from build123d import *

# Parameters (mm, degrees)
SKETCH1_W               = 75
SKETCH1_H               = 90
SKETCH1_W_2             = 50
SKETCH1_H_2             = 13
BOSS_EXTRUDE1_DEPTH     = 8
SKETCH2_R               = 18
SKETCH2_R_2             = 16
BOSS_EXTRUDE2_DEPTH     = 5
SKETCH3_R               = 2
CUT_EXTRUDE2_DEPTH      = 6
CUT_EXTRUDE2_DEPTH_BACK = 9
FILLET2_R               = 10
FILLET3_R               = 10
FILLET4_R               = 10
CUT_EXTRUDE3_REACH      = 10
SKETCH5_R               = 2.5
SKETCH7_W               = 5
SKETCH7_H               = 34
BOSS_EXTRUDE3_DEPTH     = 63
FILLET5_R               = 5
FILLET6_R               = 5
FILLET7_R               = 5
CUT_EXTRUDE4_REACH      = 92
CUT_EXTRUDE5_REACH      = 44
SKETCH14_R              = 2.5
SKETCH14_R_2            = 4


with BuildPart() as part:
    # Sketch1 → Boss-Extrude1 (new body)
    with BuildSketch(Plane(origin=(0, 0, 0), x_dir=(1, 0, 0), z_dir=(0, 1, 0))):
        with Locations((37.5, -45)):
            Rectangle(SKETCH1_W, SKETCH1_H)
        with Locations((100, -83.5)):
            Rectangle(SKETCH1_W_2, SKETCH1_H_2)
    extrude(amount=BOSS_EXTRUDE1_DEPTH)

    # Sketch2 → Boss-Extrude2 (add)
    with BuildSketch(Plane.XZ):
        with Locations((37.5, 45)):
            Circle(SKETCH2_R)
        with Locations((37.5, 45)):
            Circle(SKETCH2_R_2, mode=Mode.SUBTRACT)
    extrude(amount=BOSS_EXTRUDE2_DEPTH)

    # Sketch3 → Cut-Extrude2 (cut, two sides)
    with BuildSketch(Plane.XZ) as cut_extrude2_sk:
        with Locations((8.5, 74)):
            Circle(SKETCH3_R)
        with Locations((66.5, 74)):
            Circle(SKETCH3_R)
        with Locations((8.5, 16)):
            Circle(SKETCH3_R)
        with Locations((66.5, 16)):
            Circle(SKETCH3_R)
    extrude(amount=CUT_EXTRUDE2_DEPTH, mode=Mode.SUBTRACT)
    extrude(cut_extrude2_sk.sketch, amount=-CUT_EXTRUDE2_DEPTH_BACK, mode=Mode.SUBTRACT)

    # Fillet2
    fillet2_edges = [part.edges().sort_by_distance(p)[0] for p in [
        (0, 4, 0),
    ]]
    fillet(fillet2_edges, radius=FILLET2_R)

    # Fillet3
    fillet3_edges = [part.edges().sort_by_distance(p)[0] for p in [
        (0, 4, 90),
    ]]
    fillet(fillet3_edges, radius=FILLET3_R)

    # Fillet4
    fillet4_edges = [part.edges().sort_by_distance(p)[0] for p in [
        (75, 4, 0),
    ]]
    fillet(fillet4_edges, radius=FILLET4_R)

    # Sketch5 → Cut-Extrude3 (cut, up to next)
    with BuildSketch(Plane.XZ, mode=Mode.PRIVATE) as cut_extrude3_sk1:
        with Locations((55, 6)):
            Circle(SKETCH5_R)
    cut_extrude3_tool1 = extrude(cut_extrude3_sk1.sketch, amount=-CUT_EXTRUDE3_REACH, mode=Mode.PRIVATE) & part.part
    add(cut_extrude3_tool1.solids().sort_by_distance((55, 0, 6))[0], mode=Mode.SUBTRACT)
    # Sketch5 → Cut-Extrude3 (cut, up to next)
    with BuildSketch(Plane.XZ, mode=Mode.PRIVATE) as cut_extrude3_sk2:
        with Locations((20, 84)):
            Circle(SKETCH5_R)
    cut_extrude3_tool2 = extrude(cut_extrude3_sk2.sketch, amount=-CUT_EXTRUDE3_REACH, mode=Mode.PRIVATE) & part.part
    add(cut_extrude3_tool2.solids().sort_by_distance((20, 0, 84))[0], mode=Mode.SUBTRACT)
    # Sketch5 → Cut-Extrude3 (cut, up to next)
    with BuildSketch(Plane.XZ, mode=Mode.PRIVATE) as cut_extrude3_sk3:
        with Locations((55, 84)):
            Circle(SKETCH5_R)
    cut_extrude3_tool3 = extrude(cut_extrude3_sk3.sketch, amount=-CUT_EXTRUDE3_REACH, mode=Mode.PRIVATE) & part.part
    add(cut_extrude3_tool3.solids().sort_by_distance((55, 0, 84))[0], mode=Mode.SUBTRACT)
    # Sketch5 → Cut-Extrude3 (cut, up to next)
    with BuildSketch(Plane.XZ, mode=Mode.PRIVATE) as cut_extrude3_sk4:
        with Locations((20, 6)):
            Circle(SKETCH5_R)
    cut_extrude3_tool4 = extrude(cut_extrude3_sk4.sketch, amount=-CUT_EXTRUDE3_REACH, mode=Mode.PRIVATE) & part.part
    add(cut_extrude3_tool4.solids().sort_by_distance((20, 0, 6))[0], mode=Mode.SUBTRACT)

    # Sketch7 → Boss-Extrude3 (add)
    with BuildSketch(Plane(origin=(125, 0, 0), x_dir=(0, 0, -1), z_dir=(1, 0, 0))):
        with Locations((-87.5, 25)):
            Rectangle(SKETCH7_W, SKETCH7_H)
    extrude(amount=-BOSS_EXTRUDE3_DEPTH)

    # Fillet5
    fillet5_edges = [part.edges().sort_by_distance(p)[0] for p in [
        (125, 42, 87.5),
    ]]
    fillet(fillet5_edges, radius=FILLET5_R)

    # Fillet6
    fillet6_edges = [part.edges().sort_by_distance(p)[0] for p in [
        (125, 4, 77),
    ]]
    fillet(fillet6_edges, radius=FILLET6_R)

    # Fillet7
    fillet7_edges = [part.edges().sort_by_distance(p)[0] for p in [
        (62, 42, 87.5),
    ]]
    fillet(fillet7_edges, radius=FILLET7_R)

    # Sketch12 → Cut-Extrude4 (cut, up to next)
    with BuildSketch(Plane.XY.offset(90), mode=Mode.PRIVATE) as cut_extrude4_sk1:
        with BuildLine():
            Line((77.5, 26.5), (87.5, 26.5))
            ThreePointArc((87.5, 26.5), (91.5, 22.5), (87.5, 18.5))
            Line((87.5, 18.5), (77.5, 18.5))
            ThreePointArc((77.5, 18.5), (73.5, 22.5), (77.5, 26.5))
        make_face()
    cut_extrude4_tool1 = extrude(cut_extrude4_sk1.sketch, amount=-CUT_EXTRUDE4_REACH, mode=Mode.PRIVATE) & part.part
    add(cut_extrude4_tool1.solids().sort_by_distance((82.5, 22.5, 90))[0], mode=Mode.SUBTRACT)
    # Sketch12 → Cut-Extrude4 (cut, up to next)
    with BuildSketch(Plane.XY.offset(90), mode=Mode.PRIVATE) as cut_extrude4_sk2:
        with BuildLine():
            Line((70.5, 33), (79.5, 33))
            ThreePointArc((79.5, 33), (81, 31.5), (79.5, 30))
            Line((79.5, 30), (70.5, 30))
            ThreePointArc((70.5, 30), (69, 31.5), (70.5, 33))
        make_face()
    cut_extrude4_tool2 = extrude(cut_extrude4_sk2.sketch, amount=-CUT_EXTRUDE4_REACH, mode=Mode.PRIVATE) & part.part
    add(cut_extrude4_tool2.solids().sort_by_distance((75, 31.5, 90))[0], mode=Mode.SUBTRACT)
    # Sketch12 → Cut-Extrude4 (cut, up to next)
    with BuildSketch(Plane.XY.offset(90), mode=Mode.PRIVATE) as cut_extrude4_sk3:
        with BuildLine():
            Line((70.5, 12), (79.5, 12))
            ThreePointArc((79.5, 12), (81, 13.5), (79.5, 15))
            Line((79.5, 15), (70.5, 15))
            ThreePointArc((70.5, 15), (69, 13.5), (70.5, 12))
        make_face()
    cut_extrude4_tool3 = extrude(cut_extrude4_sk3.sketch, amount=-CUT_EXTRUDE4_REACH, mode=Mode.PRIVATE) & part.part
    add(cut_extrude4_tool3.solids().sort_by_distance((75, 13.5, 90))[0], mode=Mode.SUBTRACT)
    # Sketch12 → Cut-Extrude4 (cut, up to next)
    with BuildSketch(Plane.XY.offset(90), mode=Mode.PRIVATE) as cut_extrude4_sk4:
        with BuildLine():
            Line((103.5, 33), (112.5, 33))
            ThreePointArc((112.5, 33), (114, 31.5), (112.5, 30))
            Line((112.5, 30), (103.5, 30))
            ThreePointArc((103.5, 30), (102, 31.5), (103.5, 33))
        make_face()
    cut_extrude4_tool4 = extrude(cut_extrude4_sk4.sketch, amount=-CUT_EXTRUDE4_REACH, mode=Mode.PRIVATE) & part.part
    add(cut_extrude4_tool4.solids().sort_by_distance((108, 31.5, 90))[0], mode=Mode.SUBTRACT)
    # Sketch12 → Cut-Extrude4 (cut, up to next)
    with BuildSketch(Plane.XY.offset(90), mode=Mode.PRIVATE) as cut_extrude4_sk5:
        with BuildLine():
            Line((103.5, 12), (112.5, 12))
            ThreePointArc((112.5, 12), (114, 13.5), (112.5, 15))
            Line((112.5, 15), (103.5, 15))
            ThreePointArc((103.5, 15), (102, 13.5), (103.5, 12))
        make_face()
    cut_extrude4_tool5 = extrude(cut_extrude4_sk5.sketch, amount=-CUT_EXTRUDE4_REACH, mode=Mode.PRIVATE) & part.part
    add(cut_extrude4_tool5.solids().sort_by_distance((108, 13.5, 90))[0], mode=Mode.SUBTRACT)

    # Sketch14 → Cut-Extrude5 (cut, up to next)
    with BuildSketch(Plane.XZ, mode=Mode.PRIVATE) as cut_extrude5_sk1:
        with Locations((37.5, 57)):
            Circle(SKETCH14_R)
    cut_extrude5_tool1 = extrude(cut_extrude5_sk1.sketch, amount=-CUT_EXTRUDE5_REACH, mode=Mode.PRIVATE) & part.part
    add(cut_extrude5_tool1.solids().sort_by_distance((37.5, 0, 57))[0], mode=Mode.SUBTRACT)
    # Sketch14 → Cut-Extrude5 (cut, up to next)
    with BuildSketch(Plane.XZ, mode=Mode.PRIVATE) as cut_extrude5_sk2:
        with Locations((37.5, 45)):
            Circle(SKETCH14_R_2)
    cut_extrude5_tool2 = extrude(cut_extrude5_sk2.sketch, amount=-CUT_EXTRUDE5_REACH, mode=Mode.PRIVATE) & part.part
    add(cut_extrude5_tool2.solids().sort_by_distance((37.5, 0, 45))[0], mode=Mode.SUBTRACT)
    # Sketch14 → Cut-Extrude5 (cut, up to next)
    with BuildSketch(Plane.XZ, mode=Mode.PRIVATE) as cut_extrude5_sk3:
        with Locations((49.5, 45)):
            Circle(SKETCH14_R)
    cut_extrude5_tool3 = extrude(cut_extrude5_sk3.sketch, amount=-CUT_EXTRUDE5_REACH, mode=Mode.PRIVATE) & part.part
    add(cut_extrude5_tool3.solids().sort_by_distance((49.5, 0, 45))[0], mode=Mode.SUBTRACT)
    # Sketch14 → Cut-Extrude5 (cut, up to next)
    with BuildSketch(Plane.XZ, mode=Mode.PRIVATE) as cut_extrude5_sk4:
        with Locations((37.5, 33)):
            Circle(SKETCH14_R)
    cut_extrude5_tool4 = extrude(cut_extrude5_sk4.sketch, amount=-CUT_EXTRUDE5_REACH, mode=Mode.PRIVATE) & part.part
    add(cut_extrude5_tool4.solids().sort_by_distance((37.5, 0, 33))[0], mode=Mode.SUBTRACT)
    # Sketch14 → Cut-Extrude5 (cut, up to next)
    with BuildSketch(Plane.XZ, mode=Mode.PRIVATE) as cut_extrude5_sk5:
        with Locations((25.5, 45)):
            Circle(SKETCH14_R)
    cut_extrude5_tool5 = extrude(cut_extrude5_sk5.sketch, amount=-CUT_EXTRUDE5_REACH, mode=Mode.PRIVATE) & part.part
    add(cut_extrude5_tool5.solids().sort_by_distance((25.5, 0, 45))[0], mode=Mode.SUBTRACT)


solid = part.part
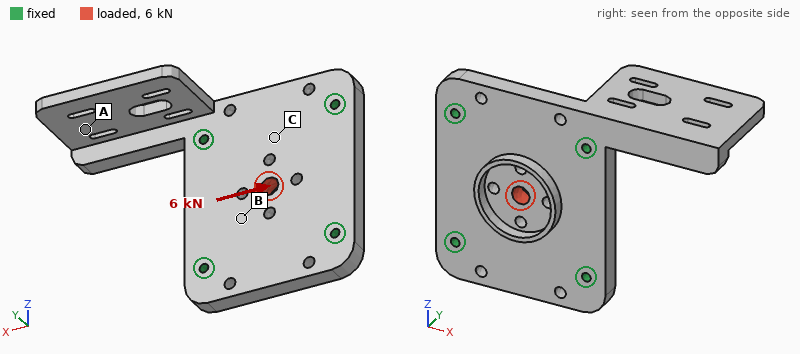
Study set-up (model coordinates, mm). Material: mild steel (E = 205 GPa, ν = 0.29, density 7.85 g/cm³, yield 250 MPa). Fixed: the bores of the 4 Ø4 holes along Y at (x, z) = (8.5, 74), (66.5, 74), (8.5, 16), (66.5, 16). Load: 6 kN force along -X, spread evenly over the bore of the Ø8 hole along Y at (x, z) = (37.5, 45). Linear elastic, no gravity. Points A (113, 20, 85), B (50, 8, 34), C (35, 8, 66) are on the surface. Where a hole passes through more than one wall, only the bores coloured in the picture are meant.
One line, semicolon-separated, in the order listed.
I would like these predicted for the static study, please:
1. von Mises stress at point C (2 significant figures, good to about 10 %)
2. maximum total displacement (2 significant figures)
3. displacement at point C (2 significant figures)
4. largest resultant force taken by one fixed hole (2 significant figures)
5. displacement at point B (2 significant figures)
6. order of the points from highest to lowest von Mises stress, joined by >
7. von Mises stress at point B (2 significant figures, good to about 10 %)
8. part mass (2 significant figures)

6.9 MPa; 3.7 µm; 1.1 µm; 1.7 kN; 1.9 µm; B > C > A; 14 MPa; 530 g
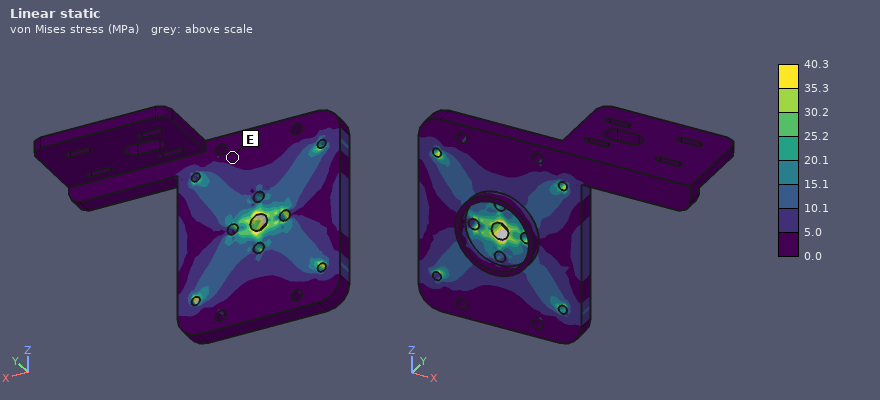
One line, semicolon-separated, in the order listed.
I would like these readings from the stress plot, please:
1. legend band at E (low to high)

0.0 to 5.0 MPa
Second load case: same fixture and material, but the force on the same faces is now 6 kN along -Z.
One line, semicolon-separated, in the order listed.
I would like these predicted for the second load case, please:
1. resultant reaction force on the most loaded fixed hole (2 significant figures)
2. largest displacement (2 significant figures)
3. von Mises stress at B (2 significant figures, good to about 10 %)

1.6 kN; 3.5 µm; 13 MPa
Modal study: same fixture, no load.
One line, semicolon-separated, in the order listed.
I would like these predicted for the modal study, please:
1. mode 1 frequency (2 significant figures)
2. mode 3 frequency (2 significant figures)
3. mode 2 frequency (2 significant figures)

1300 Hz; 2700 Hz; 1600 Hz
